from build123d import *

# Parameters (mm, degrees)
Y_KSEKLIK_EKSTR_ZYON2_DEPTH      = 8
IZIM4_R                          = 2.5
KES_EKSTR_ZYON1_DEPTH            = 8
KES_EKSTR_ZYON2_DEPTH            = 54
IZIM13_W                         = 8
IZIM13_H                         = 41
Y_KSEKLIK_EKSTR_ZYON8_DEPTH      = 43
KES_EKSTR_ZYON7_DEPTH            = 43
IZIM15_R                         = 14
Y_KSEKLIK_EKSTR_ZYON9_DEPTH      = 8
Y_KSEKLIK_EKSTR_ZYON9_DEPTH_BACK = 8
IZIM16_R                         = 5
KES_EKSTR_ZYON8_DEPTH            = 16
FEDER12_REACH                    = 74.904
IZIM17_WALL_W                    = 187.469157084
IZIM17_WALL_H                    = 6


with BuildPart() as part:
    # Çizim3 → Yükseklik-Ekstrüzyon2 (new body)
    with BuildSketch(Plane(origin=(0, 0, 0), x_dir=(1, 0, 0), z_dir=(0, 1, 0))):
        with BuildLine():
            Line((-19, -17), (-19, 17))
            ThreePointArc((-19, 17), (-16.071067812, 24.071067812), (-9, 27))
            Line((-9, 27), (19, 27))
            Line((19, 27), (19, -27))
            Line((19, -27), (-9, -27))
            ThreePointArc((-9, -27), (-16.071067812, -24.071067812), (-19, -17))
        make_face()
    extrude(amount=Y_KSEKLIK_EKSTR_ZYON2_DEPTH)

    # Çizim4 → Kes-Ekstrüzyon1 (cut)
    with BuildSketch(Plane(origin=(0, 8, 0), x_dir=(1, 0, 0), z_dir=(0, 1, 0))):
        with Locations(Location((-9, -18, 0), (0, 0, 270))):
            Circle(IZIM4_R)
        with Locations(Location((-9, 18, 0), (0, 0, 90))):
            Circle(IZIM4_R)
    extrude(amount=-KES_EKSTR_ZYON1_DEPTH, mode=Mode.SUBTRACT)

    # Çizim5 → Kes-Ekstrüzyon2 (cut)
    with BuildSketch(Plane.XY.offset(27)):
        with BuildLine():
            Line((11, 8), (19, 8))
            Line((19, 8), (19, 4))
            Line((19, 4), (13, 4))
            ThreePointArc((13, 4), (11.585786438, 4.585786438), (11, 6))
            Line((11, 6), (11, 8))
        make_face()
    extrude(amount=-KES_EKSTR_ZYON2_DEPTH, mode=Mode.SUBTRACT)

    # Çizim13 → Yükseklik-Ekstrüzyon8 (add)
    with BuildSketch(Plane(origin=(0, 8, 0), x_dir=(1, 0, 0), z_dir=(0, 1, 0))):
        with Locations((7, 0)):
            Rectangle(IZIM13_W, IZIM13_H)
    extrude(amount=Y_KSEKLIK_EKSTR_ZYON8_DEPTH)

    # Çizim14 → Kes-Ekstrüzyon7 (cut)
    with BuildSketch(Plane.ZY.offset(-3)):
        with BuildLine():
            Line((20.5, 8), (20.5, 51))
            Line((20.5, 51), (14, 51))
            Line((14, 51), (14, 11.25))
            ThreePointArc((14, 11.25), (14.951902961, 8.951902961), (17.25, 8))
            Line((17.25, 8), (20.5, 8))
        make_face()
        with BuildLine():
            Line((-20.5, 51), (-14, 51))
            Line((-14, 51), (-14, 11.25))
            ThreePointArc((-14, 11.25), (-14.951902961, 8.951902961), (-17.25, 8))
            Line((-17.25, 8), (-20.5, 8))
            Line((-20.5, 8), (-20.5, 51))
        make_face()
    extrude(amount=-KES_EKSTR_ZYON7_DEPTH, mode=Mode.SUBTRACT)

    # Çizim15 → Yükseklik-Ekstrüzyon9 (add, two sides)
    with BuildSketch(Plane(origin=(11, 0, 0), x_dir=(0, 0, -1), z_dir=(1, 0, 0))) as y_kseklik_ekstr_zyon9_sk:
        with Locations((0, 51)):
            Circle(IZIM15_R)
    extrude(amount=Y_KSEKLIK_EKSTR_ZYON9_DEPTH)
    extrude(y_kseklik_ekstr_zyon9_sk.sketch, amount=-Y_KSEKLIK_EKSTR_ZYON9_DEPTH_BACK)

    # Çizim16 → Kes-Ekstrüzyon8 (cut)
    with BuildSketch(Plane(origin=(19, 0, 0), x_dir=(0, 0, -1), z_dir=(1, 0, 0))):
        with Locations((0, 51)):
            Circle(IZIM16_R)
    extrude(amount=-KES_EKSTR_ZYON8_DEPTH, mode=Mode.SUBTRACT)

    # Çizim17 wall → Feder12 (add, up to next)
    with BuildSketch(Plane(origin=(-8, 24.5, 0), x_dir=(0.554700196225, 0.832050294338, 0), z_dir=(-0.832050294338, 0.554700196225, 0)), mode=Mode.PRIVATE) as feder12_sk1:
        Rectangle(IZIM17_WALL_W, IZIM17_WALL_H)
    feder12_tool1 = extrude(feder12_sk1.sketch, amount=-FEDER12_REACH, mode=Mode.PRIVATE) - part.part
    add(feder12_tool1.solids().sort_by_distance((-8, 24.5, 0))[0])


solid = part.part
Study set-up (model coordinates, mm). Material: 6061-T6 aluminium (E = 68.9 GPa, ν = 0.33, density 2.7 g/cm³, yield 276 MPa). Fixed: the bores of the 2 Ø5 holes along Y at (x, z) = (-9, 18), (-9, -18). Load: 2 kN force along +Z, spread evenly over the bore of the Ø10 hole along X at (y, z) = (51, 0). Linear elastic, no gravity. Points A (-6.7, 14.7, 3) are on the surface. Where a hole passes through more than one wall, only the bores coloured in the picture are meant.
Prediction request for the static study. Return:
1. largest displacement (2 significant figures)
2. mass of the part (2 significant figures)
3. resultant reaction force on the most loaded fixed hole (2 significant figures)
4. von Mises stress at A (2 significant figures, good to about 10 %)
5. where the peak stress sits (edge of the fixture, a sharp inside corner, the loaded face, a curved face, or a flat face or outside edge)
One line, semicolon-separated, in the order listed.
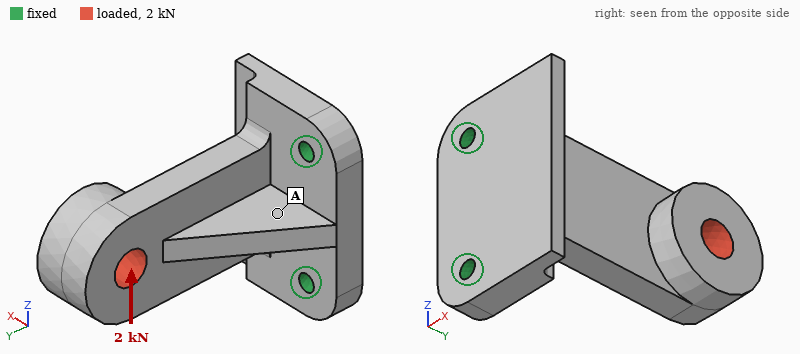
0.25 mm; 87 g; 3.1 kN; 32 MPa; a curved face
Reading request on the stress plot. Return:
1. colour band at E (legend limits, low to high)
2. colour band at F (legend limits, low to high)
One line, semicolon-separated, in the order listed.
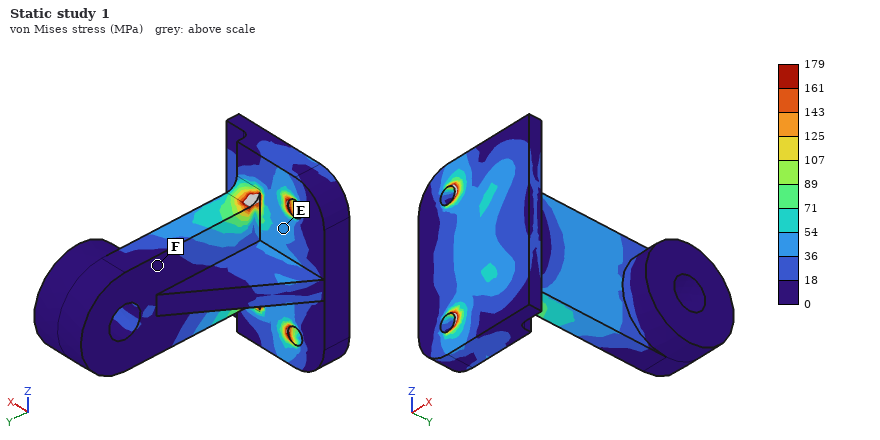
36 to 54 MPa; 0 to 18 MPa
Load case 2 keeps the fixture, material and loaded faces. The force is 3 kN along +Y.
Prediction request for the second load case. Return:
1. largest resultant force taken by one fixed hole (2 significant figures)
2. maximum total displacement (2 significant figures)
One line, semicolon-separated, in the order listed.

1.5 kN; 0.29 mm
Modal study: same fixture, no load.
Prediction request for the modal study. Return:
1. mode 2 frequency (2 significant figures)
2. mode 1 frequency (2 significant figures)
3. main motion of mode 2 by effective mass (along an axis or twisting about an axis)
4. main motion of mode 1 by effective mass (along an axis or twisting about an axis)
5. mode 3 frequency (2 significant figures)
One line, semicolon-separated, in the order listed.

3100 Hz; 2000 Hz; along Z; along X; 6700 Hz
